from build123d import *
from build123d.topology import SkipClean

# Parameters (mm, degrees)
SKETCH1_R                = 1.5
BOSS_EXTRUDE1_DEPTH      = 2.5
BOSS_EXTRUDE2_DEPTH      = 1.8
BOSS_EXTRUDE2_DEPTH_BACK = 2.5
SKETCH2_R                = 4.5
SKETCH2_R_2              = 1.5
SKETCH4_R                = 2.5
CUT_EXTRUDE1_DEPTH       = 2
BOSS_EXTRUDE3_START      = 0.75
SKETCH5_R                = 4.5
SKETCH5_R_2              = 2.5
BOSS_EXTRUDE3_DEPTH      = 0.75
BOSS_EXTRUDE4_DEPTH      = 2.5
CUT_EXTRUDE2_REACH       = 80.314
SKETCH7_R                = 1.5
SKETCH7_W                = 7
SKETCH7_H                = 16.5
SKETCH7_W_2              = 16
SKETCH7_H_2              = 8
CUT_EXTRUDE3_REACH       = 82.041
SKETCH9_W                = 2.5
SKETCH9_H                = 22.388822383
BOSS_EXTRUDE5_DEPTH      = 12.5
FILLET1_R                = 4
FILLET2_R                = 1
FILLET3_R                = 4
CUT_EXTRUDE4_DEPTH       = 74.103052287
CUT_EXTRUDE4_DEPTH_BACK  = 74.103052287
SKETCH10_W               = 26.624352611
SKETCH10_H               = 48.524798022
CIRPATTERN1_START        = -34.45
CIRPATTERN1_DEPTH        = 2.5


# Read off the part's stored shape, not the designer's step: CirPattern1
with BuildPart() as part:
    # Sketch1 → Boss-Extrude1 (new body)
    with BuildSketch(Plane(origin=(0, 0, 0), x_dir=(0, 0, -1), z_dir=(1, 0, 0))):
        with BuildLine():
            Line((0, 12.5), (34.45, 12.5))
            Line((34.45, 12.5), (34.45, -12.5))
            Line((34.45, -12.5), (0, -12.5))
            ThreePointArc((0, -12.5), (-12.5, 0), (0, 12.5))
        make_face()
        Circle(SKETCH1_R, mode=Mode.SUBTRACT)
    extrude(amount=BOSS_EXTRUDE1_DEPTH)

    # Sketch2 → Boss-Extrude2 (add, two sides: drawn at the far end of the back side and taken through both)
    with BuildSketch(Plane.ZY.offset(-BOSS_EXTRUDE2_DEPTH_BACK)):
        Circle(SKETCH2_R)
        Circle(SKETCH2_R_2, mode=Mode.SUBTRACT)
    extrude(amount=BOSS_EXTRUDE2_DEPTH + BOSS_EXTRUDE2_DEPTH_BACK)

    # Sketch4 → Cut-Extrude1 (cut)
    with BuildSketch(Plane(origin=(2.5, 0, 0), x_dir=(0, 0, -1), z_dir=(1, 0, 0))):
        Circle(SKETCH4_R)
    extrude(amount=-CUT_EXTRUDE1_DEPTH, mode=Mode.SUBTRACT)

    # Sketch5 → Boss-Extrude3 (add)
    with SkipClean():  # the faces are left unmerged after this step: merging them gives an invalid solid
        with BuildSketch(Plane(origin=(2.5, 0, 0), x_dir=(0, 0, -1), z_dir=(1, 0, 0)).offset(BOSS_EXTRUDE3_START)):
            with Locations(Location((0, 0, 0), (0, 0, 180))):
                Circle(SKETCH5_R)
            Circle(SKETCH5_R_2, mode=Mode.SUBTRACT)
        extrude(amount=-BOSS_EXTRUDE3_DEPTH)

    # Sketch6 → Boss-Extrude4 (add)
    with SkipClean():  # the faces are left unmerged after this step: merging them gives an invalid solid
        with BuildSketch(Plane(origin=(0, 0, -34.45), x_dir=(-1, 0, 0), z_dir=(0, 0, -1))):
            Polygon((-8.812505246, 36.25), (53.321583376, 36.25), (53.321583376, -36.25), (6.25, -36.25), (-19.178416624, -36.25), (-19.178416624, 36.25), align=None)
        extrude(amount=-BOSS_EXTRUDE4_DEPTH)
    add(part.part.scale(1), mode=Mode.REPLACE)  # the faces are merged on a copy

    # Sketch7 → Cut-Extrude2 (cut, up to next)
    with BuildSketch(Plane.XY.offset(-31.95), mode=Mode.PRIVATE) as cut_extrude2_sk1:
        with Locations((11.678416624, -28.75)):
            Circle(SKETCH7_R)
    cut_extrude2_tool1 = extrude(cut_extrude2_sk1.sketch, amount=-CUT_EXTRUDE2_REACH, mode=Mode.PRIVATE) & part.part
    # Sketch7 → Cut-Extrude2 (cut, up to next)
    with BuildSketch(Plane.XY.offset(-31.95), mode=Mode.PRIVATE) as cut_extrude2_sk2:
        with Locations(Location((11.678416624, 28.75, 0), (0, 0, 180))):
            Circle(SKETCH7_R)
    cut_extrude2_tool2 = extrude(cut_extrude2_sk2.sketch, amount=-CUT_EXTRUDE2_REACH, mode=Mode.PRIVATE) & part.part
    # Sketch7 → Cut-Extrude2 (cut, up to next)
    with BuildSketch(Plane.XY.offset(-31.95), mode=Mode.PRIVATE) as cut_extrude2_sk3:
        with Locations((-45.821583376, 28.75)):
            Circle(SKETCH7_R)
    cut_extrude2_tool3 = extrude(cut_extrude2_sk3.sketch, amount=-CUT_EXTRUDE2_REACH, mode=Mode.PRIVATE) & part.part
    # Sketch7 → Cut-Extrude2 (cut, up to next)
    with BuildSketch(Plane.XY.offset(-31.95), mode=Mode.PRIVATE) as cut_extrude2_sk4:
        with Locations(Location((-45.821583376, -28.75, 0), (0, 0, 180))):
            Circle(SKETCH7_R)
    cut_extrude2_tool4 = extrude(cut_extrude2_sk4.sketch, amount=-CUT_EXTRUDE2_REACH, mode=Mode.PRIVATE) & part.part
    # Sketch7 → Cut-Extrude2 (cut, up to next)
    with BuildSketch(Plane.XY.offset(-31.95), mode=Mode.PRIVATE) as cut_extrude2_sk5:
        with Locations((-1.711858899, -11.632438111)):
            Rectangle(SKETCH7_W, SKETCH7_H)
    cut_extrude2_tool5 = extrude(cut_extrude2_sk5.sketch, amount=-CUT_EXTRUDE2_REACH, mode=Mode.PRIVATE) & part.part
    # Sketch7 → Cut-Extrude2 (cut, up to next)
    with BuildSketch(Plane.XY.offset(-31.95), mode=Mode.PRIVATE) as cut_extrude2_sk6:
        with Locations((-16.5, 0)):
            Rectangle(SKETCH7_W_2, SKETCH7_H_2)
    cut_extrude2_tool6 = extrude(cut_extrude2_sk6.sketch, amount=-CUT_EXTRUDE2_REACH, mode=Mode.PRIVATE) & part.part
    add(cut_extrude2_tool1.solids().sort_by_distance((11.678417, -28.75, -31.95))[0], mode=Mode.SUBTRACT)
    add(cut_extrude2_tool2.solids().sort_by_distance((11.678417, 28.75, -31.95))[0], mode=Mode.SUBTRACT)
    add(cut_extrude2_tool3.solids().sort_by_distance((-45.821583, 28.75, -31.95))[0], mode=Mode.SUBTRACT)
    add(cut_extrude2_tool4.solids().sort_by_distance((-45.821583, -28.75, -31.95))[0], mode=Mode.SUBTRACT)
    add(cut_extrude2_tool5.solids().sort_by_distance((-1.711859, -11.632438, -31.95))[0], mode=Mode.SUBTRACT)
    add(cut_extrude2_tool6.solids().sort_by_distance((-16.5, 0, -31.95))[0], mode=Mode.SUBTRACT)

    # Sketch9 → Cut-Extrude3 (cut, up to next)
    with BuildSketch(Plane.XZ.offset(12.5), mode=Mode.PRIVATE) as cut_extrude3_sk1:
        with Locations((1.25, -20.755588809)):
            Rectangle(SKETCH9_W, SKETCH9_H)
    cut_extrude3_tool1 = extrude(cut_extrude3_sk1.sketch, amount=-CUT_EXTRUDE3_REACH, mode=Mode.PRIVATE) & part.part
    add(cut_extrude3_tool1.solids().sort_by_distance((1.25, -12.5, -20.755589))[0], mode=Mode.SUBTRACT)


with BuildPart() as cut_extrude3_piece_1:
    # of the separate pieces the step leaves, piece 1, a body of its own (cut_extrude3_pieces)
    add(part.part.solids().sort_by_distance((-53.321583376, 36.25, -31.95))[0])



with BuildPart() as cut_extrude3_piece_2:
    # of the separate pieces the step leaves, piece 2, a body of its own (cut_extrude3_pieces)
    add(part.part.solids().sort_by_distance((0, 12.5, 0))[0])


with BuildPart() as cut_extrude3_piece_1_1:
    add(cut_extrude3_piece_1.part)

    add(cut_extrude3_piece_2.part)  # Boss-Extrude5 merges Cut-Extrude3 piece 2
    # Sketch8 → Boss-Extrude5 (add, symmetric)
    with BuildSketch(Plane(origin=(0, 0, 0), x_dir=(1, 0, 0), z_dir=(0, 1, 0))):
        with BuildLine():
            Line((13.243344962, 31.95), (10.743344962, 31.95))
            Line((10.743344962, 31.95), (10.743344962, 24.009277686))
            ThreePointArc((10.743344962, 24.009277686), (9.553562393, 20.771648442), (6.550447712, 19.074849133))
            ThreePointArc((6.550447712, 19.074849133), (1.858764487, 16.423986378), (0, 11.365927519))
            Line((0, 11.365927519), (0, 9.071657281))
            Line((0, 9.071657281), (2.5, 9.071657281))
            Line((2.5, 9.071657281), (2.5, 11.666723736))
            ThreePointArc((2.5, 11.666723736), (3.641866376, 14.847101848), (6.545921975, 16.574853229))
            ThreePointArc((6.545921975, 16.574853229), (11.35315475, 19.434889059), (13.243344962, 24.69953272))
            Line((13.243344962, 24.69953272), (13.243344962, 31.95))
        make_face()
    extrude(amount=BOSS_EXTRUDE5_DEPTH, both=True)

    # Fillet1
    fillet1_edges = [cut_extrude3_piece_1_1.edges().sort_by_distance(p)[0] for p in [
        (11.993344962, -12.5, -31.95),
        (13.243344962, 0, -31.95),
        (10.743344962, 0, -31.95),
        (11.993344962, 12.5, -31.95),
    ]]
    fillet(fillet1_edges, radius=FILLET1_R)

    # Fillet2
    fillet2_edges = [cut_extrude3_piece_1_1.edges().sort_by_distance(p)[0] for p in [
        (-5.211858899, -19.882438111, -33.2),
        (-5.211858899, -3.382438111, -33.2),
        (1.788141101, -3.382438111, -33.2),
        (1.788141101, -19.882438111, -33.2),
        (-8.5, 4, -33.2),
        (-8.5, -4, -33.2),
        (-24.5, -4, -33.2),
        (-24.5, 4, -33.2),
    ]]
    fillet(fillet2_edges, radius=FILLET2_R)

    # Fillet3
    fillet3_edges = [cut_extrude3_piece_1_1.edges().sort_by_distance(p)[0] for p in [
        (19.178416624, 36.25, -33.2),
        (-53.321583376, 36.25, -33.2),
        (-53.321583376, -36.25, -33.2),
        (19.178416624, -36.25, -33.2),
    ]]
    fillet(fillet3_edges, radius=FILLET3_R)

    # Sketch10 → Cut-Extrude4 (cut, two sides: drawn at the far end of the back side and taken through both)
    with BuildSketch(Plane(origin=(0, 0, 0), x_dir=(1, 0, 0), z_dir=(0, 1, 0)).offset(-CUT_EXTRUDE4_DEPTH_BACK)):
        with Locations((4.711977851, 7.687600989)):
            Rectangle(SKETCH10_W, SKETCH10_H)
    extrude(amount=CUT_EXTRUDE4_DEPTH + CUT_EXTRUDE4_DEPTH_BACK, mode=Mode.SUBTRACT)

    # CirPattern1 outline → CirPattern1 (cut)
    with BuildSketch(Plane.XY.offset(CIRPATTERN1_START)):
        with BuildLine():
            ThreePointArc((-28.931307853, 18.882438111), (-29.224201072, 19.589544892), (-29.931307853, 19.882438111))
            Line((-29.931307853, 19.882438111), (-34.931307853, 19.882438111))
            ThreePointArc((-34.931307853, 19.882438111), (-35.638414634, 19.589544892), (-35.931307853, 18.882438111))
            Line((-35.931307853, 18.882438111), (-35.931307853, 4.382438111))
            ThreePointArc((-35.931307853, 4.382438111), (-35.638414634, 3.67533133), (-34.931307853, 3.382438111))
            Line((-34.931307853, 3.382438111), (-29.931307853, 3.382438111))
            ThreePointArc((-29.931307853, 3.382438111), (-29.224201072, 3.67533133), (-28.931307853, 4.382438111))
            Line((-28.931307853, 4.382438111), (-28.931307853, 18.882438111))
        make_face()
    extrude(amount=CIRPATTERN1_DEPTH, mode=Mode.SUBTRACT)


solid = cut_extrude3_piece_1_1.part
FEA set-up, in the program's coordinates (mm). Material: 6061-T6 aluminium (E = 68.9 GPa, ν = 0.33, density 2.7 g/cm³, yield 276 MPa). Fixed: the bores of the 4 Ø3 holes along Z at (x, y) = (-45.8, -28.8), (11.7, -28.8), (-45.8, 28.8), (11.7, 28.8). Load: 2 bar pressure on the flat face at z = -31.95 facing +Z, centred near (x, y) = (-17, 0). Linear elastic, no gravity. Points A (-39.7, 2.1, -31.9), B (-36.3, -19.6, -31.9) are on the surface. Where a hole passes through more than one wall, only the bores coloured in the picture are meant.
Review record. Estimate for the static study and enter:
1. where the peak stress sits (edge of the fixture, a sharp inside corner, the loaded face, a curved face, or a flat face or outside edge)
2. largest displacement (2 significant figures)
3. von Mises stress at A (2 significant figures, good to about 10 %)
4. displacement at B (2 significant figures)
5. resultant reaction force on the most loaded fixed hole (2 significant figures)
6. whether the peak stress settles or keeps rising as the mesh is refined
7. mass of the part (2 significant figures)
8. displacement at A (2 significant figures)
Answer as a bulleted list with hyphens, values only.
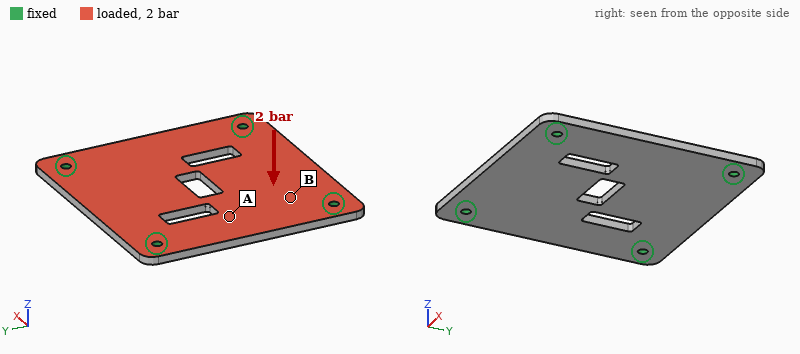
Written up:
- edge of the fixture
- 0.19 mm
- 38 MPa
- 0.066 mm
- 240 N
- keeps rising
- 33 g
- 0.11 mm
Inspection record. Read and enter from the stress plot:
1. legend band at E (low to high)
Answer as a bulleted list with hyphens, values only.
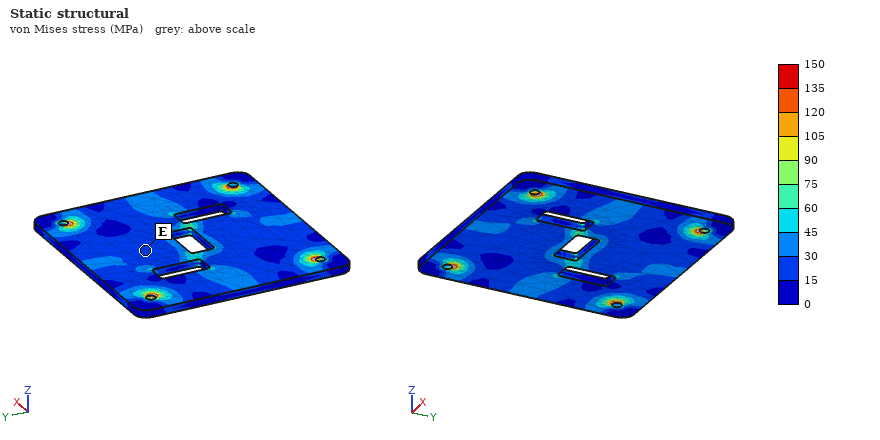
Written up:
- 15 to 30 MPa
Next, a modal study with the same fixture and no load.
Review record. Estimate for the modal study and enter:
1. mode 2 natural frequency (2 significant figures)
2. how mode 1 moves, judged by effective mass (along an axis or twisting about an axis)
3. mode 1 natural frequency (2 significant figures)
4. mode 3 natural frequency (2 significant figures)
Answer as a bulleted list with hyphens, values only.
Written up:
- 4200 Hz
- along Z
- 2600 Hz
- 4200 Hz
